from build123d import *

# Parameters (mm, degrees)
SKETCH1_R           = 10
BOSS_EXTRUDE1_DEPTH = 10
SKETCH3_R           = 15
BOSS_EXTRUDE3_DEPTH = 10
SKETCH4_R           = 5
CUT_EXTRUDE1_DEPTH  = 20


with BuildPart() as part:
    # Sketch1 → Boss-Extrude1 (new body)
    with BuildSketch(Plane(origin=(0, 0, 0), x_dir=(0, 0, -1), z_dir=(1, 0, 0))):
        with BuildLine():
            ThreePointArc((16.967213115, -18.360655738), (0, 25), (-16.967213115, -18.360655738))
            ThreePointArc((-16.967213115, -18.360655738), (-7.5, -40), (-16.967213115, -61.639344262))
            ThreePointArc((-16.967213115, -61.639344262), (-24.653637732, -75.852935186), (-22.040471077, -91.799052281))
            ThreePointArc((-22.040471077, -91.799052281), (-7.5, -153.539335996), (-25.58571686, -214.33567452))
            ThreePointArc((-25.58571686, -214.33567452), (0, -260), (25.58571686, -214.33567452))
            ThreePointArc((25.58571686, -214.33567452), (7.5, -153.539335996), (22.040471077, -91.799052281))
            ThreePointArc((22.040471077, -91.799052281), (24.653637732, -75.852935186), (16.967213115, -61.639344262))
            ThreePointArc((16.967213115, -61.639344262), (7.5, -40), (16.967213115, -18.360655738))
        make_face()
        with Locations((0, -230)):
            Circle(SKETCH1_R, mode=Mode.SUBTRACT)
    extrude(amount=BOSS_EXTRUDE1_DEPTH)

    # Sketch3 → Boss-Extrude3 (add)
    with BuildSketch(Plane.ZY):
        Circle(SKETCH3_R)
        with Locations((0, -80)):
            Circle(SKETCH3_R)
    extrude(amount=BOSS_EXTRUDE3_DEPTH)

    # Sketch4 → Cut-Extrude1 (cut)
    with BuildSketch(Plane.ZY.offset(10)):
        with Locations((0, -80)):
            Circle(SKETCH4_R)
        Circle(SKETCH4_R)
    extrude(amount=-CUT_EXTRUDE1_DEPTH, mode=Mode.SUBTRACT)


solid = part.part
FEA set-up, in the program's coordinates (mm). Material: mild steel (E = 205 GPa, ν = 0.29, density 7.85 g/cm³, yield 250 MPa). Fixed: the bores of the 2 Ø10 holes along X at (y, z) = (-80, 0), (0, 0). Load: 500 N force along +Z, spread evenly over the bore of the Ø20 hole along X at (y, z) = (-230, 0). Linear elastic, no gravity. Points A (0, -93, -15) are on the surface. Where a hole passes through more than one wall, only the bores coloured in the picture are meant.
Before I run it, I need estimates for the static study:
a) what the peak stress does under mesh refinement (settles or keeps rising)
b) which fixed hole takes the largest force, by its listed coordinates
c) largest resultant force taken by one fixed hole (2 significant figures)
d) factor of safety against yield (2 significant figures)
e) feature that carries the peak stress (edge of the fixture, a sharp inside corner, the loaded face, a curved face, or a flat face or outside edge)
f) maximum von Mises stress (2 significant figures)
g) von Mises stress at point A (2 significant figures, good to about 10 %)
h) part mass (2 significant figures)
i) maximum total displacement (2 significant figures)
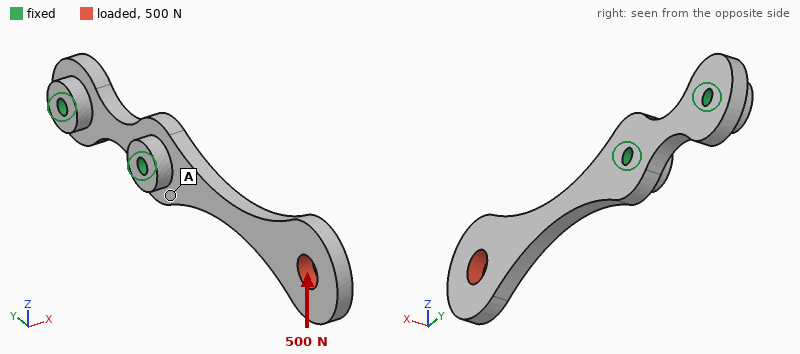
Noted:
settles
(-80, 0)
870 N
2.2
a curved face
110 MPa
19 MPa
810 g
0.44 mm
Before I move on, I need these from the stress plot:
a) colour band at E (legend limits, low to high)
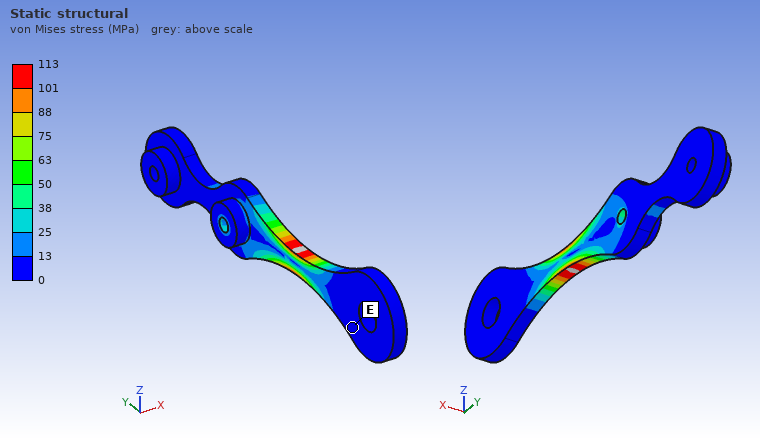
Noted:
0 to 13 MPa
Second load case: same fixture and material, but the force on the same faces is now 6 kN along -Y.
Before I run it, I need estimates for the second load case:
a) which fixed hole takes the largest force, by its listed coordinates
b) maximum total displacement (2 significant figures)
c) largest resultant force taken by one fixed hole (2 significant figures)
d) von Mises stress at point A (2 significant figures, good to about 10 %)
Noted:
(-80, 0)
24 µm
5.8 kN
8.2 MPa
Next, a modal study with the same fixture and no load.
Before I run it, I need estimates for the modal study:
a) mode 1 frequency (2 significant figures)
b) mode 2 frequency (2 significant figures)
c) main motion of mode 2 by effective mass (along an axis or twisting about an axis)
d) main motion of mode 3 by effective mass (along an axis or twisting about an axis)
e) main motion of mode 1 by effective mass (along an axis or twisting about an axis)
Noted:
210 Hz
400 Hz
along Z
twisting about Y
along X
